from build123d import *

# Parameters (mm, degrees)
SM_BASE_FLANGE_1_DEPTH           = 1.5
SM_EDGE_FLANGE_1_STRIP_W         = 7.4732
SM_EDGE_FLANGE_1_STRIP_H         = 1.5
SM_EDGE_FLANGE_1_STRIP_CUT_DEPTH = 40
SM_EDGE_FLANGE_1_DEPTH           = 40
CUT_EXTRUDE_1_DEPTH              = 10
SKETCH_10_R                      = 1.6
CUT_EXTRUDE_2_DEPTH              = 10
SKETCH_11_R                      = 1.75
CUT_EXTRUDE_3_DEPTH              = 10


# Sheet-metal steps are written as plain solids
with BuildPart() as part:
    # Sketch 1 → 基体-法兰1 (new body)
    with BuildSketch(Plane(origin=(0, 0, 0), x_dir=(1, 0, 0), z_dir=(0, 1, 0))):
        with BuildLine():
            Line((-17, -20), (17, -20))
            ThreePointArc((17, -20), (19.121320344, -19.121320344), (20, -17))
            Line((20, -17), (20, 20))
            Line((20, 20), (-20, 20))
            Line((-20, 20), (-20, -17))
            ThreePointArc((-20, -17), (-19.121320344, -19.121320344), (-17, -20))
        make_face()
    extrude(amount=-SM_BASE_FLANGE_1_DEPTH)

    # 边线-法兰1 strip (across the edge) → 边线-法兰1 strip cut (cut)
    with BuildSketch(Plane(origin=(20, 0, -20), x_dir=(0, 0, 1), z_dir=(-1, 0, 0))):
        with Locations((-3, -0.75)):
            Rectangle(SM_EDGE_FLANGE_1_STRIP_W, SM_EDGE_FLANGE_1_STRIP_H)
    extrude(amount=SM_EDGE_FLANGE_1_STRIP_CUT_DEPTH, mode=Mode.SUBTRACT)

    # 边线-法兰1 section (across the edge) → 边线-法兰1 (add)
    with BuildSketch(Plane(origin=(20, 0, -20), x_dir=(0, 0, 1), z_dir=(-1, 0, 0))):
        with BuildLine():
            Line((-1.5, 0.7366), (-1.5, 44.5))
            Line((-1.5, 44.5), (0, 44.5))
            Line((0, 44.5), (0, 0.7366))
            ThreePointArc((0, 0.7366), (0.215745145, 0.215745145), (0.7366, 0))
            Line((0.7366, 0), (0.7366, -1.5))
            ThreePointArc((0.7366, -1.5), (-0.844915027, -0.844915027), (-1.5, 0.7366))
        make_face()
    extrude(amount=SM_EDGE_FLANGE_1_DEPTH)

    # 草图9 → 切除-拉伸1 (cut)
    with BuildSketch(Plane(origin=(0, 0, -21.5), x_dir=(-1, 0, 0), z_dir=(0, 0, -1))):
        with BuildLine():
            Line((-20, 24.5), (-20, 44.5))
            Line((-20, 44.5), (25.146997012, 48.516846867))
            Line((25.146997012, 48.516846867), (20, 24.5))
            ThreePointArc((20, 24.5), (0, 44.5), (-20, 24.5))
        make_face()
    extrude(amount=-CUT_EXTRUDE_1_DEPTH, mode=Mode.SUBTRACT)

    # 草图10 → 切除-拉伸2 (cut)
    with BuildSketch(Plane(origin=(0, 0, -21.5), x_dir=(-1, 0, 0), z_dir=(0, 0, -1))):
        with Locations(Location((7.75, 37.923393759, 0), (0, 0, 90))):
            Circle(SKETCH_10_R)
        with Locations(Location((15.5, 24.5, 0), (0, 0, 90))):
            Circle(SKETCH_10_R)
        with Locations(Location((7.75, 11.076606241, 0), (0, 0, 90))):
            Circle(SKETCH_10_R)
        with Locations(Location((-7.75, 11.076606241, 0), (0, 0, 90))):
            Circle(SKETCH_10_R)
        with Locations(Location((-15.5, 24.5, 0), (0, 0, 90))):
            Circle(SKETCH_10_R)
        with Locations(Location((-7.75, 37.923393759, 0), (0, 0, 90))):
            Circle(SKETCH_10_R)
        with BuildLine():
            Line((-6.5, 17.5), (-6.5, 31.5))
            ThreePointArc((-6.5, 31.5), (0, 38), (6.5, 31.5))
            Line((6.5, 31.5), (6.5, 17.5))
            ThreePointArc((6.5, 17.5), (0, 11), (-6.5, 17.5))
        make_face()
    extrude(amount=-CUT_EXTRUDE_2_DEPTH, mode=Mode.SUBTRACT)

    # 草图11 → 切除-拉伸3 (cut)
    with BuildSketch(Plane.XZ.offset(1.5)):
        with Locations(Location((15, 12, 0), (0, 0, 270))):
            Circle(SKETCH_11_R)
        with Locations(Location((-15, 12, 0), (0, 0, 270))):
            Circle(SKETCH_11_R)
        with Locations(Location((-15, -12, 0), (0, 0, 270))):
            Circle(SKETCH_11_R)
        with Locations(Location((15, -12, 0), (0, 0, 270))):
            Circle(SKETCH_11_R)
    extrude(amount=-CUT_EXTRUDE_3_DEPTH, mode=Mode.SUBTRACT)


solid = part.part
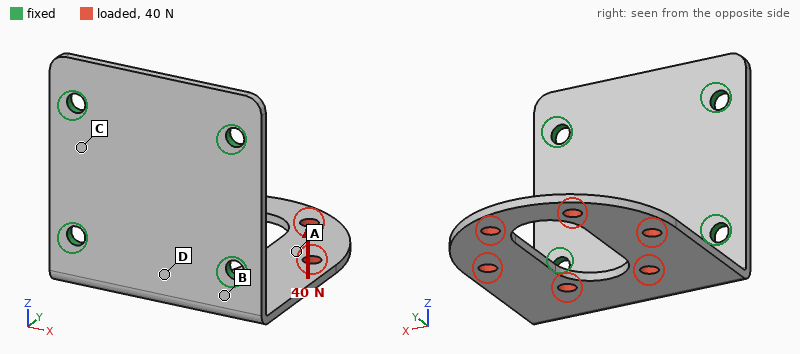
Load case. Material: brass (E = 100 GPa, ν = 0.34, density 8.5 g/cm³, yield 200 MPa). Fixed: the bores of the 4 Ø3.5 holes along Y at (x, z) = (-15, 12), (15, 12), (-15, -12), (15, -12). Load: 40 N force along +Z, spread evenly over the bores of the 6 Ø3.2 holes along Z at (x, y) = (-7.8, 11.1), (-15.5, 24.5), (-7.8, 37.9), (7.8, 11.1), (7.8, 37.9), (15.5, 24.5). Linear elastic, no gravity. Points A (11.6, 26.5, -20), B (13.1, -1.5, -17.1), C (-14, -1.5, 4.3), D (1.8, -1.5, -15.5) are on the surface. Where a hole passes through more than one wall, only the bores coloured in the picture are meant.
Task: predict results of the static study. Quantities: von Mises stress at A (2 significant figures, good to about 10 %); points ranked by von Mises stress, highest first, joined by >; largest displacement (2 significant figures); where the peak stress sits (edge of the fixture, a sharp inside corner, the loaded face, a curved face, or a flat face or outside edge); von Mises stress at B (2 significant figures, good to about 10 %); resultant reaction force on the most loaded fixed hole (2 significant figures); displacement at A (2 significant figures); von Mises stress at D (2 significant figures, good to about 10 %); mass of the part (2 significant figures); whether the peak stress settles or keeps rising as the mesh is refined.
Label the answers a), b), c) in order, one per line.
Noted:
a) 19 MPa
b) B > D > A > C
c) 0.84 mm
d) edge of the fixture
e) 66 MPa
f) 14 N
g) 0.42 mm
h) 43 MPa
i) 36 g
j) keeps rising
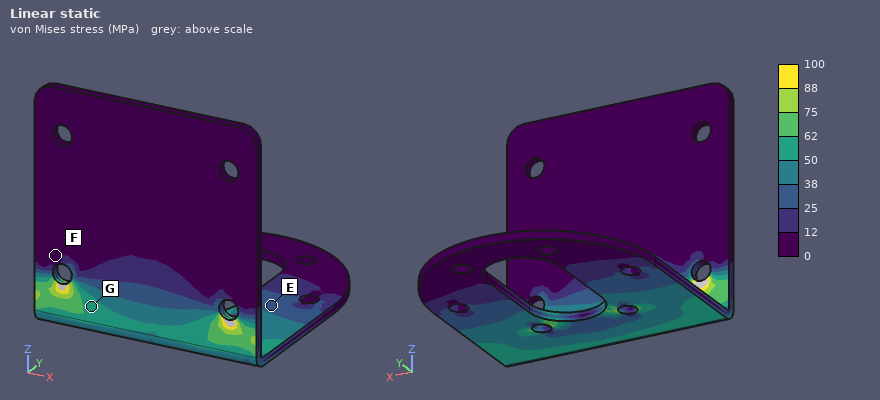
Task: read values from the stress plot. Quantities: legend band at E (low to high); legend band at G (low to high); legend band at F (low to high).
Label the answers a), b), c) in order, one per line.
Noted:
a) 25 to 38 MPa
b) 50 to 62 MPa
c) 0 to 12 MPa
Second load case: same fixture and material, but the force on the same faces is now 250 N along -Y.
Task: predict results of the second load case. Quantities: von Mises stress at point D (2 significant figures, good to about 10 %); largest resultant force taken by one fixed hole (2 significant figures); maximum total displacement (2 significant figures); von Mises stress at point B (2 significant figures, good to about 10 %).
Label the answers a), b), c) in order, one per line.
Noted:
a) 35 MPa
b) 130 N
c) 0.35 mm
d) 74 MPa
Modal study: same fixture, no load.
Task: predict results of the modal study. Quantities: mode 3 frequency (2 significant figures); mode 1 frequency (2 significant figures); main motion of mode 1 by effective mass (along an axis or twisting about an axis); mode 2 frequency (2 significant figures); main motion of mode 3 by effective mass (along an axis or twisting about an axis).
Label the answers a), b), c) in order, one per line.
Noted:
a) 2000 Hz
b) 410 Hz
c) along Z
d) 1100 Hz
e) along X
